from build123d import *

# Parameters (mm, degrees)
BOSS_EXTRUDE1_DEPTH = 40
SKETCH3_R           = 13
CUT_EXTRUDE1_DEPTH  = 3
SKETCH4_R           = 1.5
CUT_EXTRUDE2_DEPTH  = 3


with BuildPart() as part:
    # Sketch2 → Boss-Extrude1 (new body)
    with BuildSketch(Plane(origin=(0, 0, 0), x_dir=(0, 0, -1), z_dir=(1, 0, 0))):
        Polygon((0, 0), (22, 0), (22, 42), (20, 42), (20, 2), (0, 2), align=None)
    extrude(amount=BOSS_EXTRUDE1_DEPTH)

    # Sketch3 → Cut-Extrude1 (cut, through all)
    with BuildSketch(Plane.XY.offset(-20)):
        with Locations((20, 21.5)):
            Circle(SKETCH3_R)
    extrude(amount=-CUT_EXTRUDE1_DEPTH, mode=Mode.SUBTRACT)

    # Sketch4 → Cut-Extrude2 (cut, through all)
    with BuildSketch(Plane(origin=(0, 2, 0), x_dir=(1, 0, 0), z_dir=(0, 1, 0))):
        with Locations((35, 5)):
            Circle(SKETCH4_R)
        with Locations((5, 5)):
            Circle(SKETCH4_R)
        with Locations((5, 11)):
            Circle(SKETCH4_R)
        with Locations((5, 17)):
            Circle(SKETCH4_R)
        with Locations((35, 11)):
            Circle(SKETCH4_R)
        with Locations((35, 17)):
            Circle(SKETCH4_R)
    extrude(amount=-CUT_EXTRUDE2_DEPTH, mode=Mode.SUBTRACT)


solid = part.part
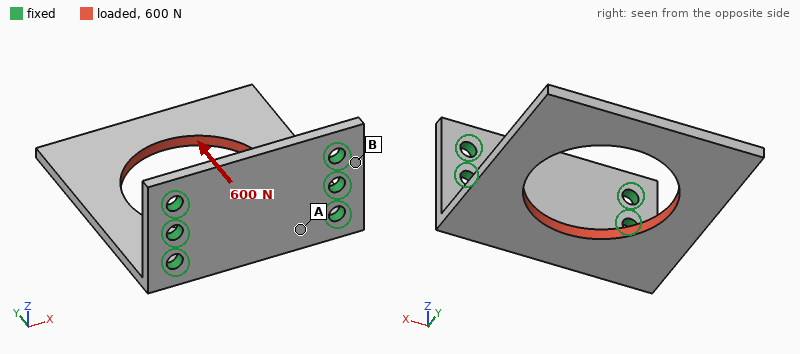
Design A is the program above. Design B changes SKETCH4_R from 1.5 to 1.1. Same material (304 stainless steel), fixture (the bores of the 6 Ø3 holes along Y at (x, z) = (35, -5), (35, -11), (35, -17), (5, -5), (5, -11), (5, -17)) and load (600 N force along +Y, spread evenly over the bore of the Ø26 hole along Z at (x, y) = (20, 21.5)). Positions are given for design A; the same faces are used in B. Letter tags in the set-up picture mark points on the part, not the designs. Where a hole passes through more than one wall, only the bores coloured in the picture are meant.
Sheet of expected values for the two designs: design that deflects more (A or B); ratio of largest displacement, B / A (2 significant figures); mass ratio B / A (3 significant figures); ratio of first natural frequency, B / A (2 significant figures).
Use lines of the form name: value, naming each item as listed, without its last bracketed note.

design that deflects more: B
ratio of largest displacement, B / A: 1.3
mass ratio B / A: 1.01
ratio of first natural frequency, B / A: 0.99
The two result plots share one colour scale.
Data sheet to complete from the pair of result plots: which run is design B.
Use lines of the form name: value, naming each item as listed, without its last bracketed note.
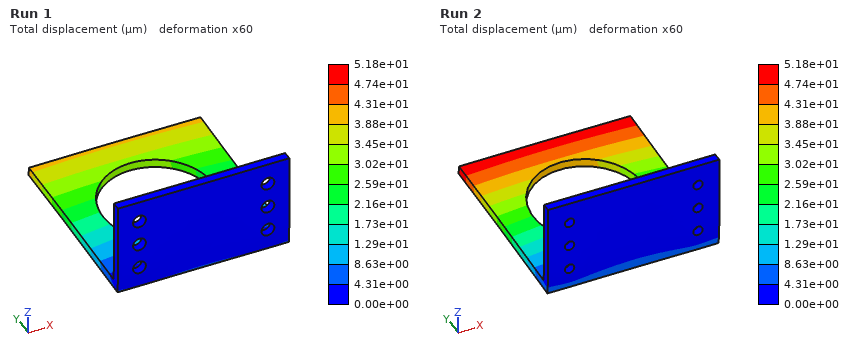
which run is design B: Run 2
